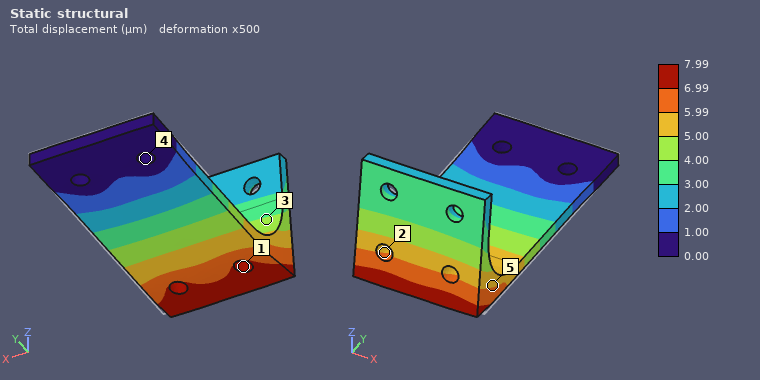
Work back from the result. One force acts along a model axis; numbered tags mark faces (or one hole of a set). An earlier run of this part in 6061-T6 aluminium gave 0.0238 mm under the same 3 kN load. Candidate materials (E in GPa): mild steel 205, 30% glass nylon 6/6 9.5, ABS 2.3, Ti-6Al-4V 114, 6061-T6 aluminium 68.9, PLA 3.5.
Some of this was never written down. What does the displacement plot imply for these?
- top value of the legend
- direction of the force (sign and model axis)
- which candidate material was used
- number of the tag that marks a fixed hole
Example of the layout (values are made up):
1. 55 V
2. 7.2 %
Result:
1. 7.99 µm
2. -Y
3. mild steel
4. 4
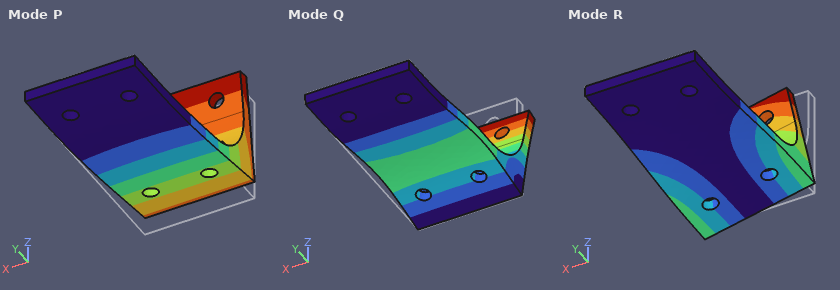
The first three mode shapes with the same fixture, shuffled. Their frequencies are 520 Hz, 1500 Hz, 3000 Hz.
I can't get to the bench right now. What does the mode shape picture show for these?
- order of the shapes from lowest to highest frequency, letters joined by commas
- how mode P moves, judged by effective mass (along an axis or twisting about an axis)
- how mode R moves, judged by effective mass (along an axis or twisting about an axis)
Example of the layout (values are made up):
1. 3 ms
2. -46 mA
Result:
1. P, R, Q
2. along Z
3. along X
